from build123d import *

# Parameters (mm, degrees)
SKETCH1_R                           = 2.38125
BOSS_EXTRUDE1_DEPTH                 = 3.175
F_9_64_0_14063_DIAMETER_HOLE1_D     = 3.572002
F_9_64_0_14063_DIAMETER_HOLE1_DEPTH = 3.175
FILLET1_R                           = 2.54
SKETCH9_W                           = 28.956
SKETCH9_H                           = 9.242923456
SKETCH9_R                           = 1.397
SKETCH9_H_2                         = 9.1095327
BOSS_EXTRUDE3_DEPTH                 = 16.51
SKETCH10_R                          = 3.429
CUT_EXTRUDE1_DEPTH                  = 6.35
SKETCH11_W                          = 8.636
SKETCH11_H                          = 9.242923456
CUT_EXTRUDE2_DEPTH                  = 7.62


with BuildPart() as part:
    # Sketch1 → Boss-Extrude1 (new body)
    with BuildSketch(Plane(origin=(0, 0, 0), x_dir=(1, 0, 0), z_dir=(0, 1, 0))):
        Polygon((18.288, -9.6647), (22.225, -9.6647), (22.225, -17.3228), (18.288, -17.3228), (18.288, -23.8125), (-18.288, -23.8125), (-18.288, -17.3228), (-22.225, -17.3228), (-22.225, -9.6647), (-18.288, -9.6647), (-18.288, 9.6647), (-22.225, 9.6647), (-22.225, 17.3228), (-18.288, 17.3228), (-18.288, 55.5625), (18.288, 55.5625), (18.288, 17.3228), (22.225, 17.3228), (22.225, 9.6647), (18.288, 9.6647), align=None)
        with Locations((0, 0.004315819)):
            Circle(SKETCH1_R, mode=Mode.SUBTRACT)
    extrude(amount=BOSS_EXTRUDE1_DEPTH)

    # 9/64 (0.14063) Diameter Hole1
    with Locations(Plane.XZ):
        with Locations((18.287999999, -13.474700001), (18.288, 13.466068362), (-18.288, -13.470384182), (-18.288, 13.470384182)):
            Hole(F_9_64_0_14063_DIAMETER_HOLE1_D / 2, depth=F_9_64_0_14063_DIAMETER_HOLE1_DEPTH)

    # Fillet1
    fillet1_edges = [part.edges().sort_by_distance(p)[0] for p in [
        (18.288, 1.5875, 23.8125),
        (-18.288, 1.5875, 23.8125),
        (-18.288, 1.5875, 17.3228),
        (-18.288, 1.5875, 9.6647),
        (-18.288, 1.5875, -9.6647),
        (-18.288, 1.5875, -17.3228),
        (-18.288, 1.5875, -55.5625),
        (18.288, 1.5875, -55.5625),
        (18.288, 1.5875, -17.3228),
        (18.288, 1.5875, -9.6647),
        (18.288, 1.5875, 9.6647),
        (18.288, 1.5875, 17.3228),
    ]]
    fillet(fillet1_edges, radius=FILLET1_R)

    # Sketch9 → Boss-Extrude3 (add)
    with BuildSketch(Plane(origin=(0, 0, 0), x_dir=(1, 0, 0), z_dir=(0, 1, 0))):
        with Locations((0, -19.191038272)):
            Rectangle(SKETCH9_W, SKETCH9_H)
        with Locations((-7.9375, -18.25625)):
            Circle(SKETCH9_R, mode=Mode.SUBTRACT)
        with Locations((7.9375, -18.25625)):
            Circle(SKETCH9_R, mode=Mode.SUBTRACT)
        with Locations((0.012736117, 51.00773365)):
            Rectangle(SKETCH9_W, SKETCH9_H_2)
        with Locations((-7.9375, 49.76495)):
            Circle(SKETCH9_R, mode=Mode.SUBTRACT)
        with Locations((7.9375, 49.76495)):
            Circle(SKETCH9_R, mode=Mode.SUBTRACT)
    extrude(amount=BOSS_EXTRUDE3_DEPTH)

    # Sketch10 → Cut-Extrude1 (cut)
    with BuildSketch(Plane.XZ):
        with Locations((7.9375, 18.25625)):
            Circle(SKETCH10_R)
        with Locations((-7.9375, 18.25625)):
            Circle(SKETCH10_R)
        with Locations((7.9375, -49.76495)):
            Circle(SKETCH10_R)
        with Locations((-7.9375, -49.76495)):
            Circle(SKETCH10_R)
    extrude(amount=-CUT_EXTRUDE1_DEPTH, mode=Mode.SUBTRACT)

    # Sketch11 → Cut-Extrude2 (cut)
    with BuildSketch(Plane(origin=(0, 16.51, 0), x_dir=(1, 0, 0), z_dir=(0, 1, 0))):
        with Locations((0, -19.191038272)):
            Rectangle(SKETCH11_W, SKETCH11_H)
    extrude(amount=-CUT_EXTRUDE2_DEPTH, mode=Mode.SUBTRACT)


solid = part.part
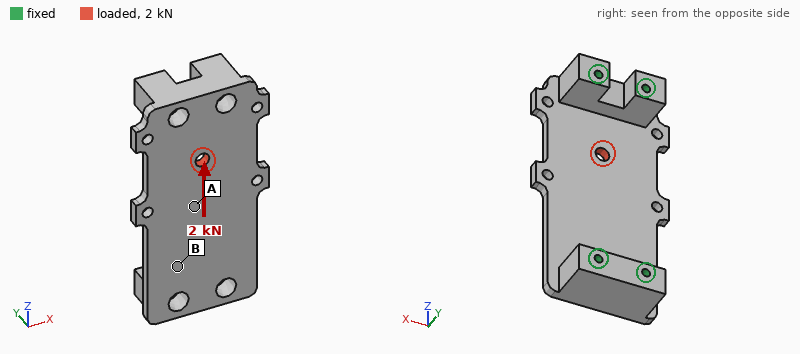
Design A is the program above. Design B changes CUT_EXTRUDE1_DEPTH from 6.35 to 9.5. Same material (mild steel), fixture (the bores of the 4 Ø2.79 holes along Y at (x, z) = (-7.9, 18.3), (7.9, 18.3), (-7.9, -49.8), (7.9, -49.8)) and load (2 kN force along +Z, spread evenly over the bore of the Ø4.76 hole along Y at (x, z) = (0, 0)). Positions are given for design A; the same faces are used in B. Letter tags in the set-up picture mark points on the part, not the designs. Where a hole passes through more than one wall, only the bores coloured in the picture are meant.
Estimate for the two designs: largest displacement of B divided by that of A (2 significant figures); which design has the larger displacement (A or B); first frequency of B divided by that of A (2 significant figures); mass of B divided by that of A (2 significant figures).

1.6
B
0.99
0.97
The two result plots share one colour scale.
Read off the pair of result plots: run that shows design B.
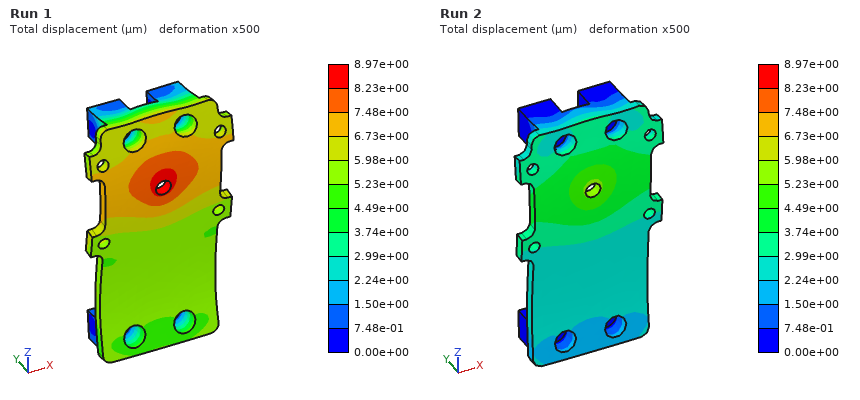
Run 1
